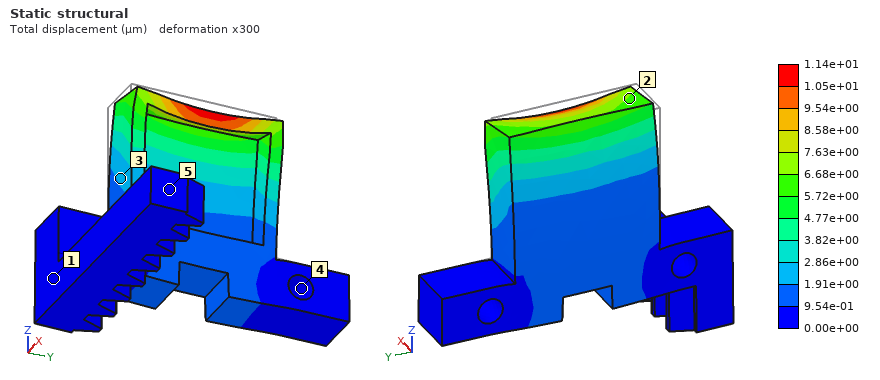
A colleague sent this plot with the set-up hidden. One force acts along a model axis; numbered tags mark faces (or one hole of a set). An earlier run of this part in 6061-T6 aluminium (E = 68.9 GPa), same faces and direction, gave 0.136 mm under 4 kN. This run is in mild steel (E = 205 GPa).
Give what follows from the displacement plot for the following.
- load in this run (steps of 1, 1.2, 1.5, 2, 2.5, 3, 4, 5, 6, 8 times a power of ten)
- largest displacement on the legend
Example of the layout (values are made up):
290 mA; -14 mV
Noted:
1 kN; 1.14e+01 µm
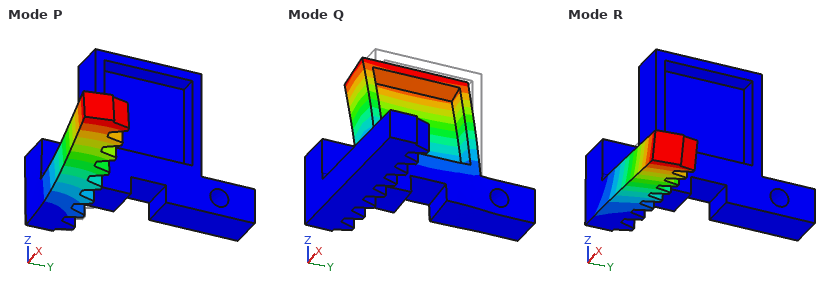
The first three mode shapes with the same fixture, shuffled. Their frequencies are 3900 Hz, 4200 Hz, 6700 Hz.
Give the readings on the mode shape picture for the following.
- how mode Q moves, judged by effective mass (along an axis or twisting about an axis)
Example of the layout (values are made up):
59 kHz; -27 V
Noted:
along X
